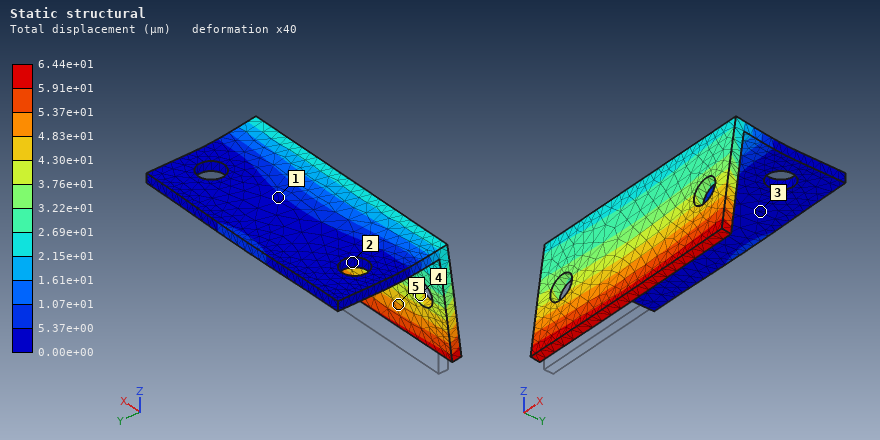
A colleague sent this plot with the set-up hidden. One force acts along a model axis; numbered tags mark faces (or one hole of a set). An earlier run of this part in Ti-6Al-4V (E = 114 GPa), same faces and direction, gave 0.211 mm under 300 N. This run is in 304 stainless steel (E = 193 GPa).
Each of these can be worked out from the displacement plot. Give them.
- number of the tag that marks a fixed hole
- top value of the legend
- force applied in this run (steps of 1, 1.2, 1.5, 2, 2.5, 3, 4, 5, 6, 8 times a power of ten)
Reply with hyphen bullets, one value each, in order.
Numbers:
- 2
- 6.44e+01 µm
- 150 N
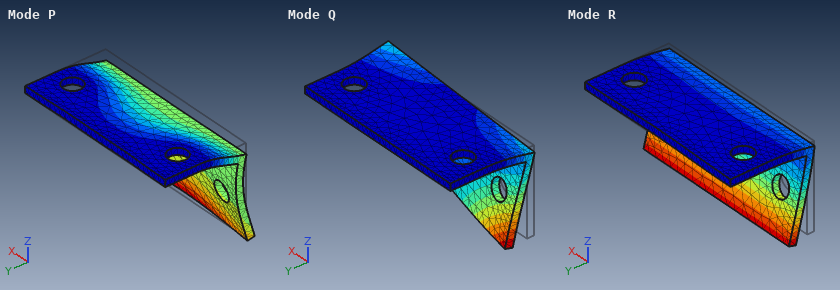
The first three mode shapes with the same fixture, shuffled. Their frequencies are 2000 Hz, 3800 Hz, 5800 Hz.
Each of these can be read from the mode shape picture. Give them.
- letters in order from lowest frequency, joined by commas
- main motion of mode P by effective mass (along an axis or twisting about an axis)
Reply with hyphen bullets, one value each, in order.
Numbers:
- R, Q, P
- along Z
